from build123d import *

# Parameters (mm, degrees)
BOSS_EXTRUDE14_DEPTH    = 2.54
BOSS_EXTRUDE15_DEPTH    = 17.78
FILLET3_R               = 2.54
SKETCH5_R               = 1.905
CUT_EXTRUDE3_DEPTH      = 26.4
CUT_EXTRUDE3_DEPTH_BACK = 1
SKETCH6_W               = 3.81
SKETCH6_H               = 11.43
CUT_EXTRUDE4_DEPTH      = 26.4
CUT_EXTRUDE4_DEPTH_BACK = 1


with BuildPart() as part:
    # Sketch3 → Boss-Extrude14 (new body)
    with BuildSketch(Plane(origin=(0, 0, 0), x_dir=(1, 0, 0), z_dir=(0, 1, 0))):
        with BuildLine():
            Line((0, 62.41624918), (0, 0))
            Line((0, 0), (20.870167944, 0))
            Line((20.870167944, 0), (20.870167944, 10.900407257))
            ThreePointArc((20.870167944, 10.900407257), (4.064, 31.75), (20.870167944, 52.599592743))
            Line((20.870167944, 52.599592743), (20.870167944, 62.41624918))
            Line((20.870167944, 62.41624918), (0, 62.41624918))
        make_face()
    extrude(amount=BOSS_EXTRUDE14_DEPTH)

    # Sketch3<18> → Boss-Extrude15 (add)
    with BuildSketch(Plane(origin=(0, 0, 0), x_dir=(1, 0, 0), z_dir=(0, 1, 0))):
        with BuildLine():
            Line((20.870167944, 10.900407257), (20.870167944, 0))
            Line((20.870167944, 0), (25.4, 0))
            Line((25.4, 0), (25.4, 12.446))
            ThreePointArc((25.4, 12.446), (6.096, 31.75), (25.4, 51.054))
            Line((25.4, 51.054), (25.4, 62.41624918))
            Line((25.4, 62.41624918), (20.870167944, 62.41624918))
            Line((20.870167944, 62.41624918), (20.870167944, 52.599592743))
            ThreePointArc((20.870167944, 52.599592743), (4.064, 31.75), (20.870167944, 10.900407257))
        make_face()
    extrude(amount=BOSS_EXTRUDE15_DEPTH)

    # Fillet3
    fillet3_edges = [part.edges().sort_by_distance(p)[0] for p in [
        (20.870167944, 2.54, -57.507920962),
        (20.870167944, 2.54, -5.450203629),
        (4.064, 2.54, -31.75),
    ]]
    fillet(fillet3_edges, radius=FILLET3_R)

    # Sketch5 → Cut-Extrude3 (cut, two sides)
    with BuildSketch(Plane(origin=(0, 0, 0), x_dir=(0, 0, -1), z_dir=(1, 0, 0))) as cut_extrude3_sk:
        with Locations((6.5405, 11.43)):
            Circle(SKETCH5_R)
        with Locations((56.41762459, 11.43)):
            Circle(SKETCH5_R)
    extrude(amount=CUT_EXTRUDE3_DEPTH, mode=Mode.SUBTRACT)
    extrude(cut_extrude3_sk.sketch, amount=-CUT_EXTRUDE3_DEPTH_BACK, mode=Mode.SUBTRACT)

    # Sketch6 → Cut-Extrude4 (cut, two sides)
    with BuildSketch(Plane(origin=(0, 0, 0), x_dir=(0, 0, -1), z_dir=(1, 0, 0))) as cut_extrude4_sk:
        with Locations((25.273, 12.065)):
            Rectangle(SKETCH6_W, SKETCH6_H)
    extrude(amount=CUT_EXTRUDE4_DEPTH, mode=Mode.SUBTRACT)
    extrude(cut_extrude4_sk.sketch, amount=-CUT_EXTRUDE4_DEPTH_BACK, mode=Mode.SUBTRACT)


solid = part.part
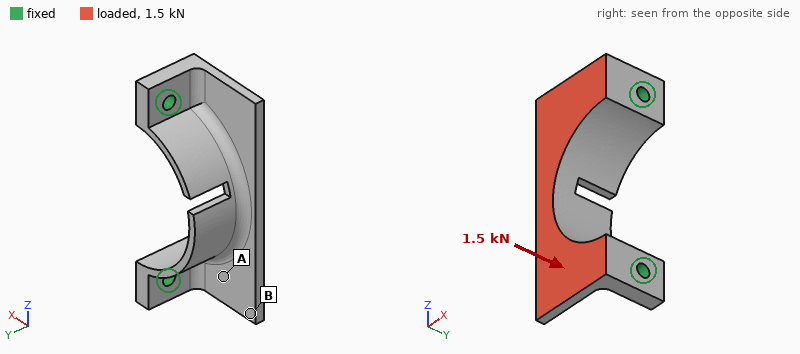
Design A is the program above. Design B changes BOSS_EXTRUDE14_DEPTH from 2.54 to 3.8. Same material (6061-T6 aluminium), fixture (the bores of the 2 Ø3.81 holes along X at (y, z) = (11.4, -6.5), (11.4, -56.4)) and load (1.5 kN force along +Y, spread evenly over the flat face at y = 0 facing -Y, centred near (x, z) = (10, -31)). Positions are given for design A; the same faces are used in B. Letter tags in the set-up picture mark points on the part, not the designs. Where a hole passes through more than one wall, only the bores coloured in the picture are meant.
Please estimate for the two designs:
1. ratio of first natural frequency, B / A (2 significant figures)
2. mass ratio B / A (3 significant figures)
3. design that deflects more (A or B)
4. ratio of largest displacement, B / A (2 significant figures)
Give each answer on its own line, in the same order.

0.93
1.17
A
0.65
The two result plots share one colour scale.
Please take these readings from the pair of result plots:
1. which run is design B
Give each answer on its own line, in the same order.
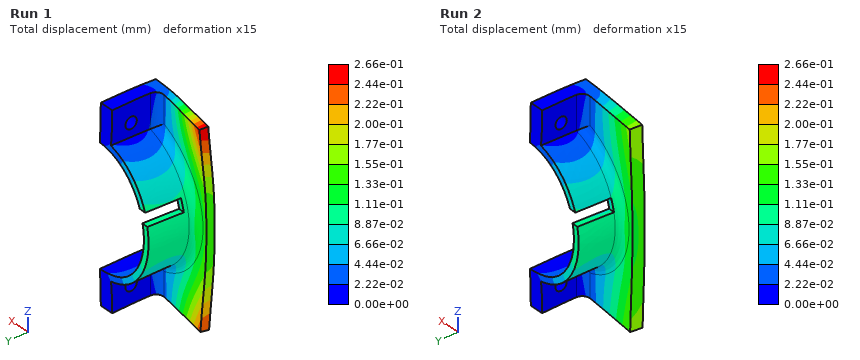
Run 2
